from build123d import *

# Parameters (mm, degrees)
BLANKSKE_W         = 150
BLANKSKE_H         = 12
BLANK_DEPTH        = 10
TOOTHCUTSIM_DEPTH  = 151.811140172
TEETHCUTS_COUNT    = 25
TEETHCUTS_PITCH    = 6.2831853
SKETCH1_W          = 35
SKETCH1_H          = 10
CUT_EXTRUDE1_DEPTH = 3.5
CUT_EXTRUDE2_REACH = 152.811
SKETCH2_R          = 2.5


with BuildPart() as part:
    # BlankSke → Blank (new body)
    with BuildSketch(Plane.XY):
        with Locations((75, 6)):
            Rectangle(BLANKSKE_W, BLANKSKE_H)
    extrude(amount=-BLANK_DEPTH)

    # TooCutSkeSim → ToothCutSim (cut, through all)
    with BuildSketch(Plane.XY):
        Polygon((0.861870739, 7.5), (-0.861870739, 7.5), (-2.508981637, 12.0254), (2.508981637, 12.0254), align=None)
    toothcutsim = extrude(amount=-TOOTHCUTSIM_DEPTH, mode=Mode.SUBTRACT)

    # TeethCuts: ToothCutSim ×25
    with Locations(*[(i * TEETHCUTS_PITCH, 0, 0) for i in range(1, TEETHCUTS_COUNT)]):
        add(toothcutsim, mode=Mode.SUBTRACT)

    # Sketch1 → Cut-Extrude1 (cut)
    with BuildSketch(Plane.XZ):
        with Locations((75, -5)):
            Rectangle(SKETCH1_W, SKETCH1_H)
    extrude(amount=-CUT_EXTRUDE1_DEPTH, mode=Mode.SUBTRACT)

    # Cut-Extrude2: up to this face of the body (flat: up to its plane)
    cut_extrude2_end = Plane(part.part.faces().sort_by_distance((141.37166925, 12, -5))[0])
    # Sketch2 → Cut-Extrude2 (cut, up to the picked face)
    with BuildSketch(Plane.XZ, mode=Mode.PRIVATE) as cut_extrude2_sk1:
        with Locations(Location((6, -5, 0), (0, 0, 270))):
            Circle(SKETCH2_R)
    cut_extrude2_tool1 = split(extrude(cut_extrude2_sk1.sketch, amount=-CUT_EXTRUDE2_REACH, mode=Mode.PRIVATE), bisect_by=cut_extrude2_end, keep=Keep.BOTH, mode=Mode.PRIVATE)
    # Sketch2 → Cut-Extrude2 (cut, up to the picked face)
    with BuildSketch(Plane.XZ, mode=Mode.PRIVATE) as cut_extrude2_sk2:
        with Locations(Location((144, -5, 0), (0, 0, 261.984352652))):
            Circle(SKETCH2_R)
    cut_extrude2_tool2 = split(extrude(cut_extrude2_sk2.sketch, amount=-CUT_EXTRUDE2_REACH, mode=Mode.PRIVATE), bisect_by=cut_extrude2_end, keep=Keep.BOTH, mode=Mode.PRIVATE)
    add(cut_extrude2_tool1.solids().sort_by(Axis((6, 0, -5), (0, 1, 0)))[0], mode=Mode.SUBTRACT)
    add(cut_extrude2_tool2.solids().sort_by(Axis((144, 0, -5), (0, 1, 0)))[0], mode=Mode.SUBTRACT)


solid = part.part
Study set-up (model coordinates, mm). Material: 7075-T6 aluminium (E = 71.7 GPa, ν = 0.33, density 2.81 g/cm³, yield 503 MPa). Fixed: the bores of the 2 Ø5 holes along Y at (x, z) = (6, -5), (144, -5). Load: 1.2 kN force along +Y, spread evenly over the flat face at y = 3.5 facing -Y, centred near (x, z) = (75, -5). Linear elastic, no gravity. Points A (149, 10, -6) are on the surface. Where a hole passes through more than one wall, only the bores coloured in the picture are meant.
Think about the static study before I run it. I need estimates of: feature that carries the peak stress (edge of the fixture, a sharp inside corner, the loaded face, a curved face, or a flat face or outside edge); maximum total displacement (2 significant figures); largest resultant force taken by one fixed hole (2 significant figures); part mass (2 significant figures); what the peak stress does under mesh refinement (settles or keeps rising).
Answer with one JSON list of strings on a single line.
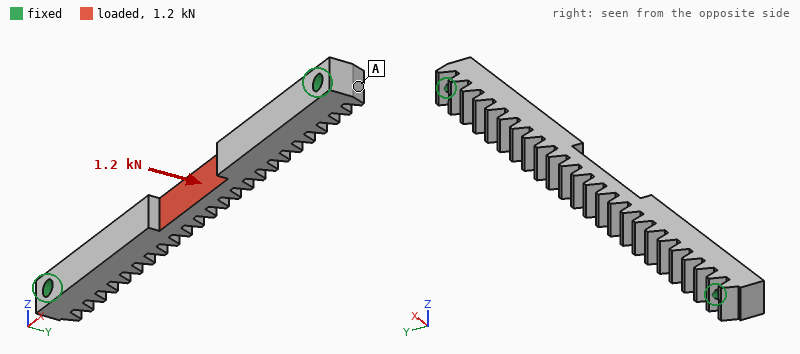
["edge of the fixture", "0.82 mm", "2.1 kN", "36 g", "keeps rising"]
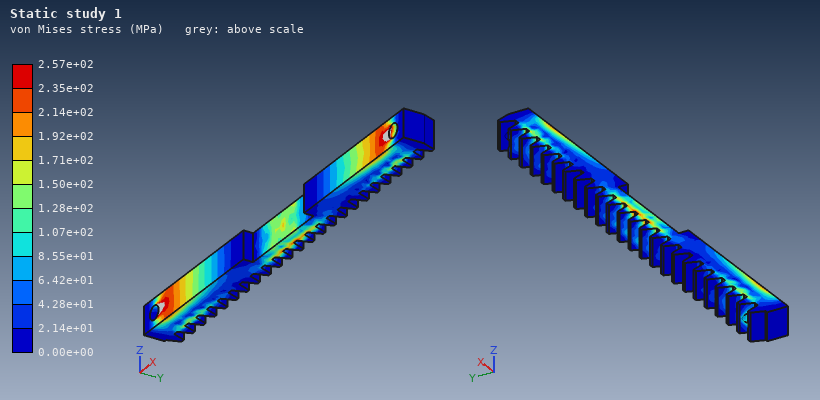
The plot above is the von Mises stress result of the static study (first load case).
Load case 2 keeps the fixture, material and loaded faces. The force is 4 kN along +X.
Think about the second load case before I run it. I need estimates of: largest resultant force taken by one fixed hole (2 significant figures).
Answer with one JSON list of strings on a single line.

["2.0 kN"]
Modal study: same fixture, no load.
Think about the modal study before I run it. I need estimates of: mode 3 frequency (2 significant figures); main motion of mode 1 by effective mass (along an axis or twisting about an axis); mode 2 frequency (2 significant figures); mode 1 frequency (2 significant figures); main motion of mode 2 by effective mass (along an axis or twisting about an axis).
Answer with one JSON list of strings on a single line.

["4300 Hz", "along Y", "2400 Hz", "1900 Hz", "along Z"]
